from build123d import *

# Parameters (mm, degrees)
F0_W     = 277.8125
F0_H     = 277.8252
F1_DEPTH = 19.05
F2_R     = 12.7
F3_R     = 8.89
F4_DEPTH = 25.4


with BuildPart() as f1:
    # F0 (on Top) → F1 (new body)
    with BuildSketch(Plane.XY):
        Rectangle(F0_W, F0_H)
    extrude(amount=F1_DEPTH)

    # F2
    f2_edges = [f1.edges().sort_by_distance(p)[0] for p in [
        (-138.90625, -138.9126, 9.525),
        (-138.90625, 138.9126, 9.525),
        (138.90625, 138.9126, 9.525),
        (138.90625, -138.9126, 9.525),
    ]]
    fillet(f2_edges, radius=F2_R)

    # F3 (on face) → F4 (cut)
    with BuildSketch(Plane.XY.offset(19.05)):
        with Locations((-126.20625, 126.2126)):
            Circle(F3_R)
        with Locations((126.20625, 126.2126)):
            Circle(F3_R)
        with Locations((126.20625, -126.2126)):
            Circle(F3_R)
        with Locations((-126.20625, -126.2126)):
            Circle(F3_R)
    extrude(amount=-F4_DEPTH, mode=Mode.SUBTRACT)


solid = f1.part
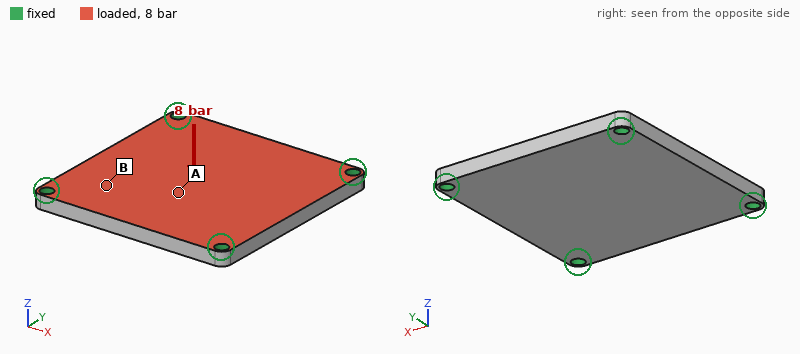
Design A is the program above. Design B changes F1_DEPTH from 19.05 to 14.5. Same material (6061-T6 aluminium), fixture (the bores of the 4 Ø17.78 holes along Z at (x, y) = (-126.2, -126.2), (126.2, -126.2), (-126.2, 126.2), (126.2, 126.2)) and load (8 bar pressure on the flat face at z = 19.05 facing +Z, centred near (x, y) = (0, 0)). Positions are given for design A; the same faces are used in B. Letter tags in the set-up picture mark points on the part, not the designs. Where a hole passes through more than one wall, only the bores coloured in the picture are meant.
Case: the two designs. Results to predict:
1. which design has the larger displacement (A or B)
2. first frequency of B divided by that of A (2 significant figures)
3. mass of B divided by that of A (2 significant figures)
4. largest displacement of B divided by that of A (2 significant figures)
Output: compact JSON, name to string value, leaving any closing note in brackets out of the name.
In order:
{"which design has the larger displacement": "B", "first frequency of B divided by that of A": "0.78", "mass of B divided by that of A": "0.76", "largest displacement of B divided by that of A": "2.2"}
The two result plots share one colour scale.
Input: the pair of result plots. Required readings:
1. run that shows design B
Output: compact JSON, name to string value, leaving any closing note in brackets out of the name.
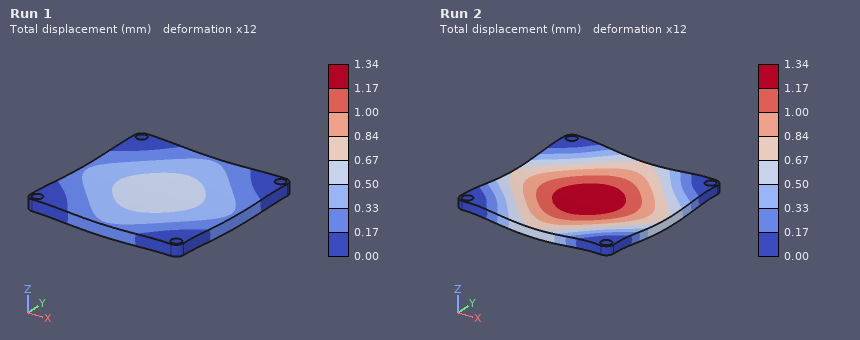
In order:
{"run that shows design B": "Run 2"}
